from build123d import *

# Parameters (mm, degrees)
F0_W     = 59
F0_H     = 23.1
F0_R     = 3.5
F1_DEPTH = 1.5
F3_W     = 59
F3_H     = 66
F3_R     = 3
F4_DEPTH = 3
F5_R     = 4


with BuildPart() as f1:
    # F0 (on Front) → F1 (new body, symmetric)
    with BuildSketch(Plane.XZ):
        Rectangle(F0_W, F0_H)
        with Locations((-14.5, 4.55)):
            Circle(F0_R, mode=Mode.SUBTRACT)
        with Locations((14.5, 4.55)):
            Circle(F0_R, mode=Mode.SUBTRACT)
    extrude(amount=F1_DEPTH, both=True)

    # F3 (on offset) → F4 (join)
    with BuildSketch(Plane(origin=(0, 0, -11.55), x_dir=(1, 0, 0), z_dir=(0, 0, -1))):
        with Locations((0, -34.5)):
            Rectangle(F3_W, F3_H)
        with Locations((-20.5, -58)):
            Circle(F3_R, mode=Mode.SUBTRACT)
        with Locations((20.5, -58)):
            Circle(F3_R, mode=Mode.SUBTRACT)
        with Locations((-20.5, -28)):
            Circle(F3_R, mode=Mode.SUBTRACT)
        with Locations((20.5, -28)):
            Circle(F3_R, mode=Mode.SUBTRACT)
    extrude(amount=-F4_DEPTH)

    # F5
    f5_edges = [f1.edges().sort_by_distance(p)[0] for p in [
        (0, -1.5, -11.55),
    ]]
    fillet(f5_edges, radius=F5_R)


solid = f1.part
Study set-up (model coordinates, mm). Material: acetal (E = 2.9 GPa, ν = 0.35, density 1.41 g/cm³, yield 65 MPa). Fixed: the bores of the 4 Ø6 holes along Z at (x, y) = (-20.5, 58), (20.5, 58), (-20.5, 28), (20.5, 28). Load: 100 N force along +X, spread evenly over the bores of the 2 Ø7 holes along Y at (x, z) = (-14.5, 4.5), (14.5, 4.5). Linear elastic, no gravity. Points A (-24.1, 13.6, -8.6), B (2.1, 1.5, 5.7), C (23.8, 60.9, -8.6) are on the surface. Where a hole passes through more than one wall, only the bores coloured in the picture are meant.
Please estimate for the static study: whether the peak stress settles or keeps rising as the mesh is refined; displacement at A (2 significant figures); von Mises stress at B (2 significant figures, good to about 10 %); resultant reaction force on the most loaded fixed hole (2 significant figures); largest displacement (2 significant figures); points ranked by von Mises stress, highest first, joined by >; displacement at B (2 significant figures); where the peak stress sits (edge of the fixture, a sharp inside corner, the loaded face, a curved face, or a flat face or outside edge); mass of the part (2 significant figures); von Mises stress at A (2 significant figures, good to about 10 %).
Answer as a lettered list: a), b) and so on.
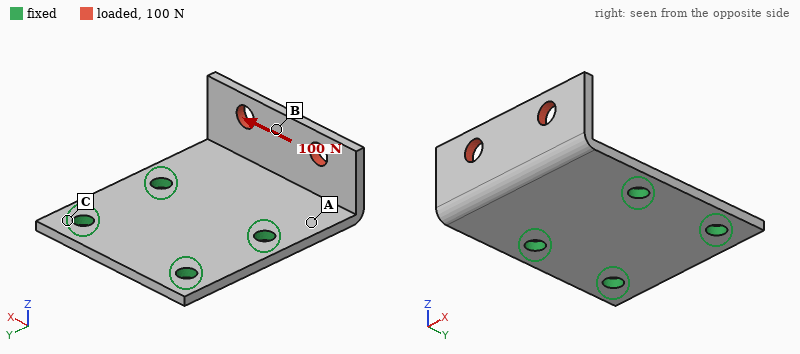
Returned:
a) keeps rising
b) 0.23 mm
c) 4.0 MPa
d) 82 N
e) 1.1 mm
f) A > B > C
g) 0.46 mm
h) edge of the fixture
i) 21 g
j) 7.1 MPa
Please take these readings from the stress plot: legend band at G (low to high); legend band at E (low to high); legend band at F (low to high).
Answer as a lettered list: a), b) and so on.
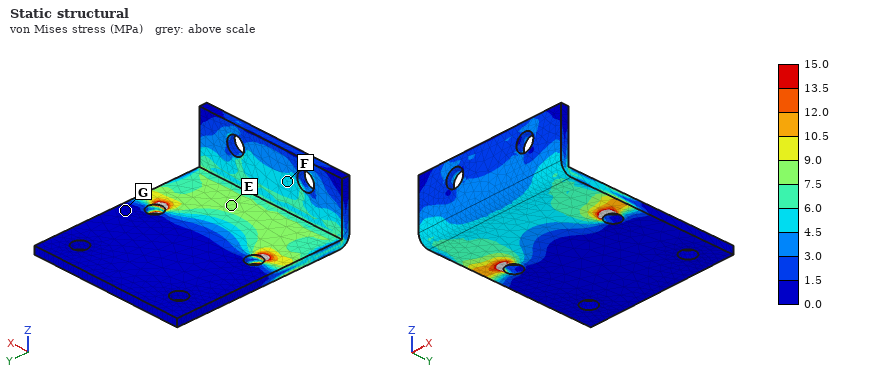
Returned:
a) 0.0 to 1.5 MPa
b) 7.5 to 9.0 MPa
c) 4.5 to 6.0 MPa
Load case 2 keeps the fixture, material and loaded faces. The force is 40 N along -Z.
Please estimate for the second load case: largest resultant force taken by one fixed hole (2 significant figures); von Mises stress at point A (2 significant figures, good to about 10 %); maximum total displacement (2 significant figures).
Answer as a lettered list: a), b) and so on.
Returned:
a) 23 N
b) 6.2 MPa
c) 1.1 mm
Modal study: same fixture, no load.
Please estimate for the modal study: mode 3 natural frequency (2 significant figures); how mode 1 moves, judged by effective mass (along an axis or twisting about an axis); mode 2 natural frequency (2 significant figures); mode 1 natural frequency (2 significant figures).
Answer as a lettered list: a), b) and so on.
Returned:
a) 1200 Hz
b) along Z
c) 690 Hz
d) 400 Hz
